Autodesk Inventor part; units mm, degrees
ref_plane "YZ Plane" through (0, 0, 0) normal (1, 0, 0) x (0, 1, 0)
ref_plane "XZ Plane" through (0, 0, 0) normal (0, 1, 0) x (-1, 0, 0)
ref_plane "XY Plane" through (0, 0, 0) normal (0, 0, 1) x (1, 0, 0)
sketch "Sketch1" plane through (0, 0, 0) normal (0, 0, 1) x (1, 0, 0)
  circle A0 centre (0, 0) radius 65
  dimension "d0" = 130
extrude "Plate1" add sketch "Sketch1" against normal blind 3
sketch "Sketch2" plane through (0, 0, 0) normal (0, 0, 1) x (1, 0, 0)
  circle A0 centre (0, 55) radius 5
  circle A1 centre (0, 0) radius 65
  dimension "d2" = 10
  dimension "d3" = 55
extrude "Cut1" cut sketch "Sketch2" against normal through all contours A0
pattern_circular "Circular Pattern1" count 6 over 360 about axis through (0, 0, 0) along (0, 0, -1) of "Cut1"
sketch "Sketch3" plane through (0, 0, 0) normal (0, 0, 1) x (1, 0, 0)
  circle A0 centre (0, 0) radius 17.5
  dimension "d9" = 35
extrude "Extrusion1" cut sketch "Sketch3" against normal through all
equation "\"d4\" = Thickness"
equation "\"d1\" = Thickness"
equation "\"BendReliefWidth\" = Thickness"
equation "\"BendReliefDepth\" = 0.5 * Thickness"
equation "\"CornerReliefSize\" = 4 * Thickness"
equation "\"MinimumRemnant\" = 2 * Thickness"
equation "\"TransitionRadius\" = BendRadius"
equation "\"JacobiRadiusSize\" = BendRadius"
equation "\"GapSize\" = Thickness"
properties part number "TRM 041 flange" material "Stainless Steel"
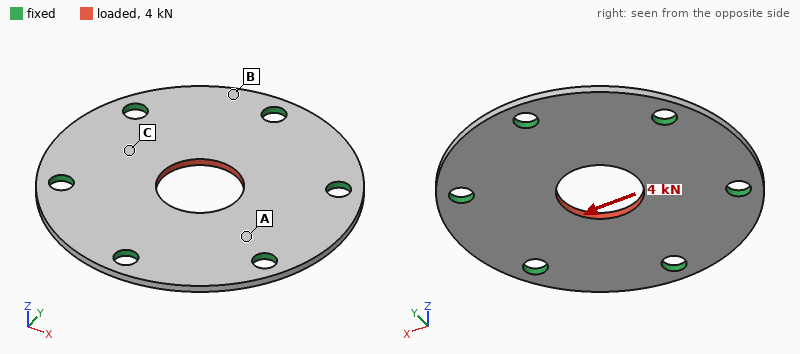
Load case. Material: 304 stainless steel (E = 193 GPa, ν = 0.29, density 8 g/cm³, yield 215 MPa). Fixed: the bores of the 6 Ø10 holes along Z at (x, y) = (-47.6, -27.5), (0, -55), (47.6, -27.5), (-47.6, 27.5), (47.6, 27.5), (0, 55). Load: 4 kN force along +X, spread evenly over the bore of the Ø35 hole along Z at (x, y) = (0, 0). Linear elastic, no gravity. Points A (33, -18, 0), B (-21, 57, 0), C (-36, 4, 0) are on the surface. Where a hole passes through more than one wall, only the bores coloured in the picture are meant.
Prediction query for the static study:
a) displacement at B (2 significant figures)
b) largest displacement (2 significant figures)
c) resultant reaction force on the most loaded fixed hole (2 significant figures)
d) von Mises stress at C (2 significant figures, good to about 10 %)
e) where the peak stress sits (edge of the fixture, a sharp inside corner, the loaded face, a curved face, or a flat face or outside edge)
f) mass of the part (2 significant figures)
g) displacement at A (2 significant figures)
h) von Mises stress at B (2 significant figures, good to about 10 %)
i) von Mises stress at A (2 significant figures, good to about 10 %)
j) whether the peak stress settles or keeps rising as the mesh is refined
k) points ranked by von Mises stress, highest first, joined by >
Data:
0.38 µm
2.4 µm
880 N
6.6 MPa
edge of the fixture
280 g
0.99 µm
2.1 MPa
12 MPa
keeps rising
A > C > B
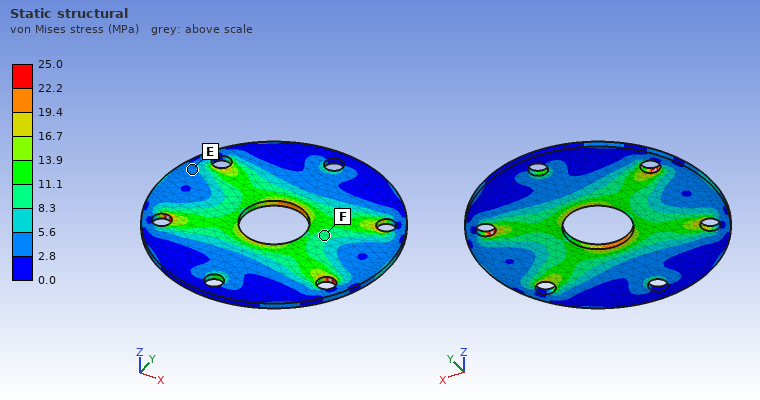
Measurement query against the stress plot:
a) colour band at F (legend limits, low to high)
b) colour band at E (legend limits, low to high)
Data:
8.3 to 11.1 MPa
2.8 to 5.6 MPa
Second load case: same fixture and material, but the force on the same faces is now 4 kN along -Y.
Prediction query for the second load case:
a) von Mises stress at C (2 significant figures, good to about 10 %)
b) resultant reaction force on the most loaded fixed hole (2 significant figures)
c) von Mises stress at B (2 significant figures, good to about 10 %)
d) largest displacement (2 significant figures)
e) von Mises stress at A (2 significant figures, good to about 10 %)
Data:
5.9 MPa
1.0 kN
3.5 MPa
2.4 µm
7.8 MPa
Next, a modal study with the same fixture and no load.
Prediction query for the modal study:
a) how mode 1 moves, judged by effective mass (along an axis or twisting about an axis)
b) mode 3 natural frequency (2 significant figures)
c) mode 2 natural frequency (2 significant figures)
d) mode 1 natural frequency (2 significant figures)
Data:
along Z
4300 Hz
4300 Hz
2700 Hz
